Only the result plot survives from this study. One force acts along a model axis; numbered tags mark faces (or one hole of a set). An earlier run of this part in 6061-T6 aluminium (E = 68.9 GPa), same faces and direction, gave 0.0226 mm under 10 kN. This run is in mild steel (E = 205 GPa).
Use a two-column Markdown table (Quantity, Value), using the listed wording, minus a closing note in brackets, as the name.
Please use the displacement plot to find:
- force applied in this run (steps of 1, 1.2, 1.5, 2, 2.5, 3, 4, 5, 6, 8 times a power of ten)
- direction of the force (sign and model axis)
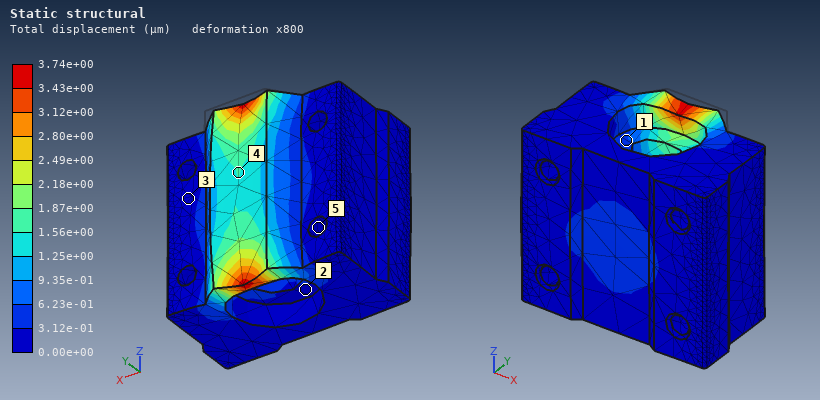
| Quantity | Value |
|---|---|
| force applied in this run | 5 kN |
| direction of the force | -Y |
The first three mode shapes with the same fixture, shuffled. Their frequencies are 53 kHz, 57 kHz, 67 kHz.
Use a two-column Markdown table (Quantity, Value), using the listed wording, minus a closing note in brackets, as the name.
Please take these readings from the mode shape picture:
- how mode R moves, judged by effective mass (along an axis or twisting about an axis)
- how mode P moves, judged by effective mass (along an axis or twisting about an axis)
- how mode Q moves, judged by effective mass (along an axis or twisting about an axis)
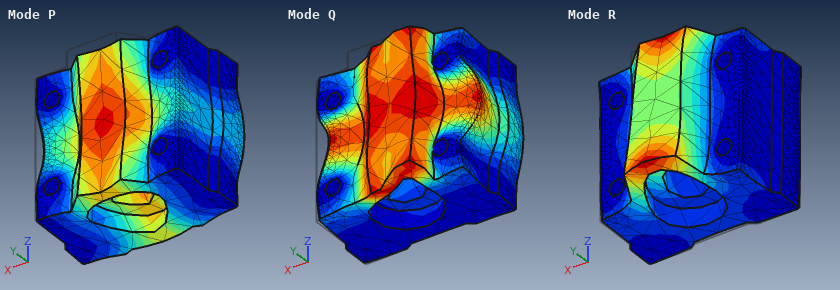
| Quantity | Value |
|---|---|
| how mode R moves, judged by effective mass | along Z |
| how mode P moves, judged by effective mass | along Y |
| how mode Q moves, judged by effective mass | along X |
